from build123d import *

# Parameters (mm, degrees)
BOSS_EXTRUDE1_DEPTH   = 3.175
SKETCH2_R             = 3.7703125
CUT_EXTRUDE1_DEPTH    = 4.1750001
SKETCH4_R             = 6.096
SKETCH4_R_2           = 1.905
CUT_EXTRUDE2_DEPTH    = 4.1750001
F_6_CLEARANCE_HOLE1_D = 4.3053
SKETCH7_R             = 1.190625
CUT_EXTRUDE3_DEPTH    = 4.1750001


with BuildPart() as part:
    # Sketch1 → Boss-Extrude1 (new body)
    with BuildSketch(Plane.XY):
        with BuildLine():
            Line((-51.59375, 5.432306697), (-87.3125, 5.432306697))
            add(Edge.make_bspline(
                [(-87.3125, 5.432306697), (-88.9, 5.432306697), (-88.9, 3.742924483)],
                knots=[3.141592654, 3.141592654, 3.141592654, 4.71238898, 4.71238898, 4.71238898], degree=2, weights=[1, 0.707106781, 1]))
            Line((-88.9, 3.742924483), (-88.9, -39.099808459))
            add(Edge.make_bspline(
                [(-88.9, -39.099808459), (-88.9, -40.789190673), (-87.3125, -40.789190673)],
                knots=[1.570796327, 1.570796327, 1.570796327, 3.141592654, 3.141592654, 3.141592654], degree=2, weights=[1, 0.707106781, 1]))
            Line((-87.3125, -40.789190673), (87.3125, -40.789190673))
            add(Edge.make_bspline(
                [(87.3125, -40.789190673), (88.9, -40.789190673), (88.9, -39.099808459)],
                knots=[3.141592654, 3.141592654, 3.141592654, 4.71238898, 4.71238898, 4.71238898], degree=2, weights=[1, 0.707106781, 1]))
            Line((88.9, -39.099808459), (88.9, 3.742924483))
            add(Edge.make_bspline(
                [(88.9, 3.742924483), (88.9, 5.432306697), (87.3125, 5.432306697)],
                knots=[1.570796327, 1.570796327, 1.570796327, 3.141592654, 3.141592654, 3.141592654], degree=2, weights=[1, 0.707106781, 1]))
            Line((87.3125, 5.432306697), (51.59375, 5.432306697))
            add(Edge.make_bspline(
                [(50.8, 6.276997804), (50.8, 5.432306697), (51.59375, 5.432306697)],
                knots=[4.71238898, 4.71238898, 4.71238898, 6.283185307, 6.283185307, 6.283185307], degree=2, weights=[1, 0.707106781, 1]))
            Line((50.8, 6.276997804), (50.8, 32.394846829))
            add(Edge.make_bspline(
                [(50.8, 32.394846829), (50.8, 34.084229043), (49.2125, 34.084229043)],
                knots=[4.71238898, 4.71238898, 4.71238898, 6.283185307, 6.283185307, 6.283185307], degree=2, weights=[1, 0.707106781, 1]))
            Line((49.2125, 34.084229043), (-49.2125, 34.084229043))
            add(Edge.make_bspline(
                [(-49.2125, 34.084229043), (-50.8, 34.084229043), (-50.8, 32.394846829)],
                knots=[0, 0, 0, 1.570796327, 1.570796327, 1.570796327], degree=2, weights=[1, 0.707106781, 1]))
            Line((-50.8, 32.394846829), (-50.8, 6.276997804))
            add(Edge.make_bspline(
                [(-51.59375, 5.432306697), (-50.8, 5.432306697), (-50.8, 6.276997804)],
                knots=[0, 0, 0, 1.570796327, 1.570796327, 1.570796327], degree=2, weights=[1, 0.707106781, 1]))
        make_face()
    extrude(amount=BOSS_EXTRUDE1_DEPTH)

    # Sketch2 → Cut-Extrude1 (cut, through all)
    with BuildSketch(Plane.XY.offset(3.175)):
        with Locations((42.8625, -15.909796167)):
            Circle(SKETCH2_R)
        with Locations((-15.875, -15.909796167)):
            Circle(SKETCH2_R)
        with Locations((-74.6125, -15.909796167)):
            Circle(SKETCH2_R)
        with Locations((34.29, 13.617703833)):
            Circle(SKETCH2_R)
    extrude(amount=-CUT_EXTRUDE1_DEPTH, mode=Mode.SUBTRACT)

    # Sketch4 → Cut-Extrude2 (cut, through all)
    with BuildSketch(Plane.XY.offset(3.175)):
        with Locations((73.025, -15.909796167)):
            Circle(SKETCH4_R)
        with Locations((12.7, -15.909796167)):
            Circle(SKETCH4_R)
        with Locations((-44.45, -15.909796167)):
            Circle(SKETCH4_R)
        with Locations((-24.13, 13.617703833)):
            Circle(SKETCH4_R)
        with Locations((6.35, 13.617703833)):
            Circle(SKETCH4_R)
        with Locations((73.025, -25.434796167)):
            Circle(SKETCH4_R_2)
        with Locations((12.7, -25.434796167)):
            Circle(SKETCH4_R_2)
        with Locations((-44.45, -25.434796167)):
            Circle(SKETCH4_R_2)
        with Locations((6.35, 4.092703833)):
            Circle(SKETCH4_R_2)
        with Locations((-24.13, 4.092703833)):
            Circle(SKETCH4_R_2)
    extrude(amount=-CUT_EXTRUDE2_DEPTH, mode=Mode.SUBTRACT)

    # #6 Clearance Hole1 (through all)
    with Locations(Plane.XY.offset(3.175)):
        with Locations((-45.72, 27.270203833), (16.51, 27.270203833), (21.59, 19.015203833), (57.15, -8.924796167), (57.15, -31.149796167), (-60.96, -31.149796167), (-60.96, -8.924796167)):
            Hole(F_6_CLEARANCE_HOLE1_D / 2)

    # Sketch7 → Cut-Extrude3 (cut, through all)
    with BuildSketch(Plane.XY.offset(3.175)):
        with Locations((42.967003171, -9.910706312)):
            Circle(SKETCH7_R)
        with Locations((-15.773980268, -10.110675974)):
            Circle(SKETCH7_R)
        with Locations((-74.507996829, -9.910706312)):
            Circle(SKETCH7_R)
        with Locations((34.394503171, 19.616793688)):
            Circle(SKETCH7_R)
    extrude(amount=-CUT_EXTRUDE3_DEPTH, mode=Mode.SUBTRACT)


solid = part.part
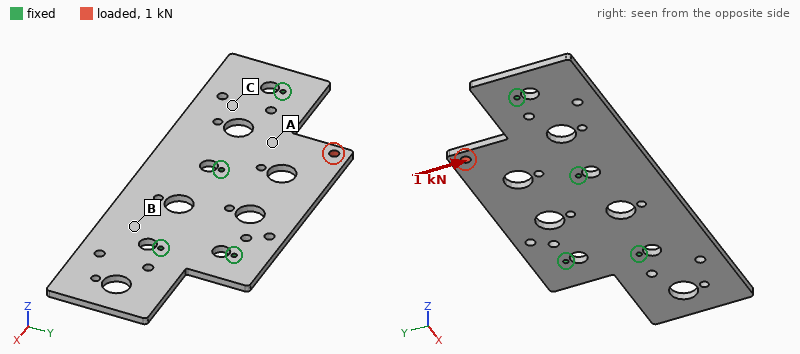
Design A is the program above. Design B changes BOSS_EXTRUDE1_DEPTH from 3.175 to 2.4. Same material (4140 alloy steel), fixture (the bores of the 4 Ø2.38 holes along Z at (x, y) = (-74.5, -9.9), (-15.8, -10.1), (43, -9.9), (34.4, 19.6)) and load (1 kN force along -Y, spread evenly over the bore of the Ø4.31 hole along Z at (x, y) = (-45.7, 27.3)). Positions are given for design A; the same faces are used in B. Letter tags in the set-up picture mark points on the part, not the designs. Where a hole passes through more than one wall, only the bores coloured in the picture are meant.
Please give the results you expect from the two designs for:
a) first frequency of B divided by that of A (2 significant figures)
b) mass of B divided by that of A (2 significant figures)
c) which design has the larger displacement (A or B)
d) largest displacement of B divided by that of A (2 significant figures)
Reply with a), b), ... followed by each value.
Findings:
a) 0.77
b) 0.76
c) B
d) 1.3
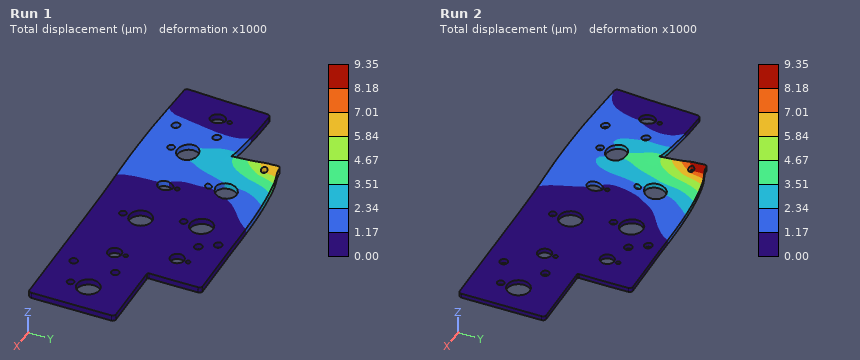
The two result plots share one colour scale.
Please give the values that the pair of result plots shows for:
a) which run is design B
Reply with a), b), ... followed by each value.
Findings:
a) Run 2
